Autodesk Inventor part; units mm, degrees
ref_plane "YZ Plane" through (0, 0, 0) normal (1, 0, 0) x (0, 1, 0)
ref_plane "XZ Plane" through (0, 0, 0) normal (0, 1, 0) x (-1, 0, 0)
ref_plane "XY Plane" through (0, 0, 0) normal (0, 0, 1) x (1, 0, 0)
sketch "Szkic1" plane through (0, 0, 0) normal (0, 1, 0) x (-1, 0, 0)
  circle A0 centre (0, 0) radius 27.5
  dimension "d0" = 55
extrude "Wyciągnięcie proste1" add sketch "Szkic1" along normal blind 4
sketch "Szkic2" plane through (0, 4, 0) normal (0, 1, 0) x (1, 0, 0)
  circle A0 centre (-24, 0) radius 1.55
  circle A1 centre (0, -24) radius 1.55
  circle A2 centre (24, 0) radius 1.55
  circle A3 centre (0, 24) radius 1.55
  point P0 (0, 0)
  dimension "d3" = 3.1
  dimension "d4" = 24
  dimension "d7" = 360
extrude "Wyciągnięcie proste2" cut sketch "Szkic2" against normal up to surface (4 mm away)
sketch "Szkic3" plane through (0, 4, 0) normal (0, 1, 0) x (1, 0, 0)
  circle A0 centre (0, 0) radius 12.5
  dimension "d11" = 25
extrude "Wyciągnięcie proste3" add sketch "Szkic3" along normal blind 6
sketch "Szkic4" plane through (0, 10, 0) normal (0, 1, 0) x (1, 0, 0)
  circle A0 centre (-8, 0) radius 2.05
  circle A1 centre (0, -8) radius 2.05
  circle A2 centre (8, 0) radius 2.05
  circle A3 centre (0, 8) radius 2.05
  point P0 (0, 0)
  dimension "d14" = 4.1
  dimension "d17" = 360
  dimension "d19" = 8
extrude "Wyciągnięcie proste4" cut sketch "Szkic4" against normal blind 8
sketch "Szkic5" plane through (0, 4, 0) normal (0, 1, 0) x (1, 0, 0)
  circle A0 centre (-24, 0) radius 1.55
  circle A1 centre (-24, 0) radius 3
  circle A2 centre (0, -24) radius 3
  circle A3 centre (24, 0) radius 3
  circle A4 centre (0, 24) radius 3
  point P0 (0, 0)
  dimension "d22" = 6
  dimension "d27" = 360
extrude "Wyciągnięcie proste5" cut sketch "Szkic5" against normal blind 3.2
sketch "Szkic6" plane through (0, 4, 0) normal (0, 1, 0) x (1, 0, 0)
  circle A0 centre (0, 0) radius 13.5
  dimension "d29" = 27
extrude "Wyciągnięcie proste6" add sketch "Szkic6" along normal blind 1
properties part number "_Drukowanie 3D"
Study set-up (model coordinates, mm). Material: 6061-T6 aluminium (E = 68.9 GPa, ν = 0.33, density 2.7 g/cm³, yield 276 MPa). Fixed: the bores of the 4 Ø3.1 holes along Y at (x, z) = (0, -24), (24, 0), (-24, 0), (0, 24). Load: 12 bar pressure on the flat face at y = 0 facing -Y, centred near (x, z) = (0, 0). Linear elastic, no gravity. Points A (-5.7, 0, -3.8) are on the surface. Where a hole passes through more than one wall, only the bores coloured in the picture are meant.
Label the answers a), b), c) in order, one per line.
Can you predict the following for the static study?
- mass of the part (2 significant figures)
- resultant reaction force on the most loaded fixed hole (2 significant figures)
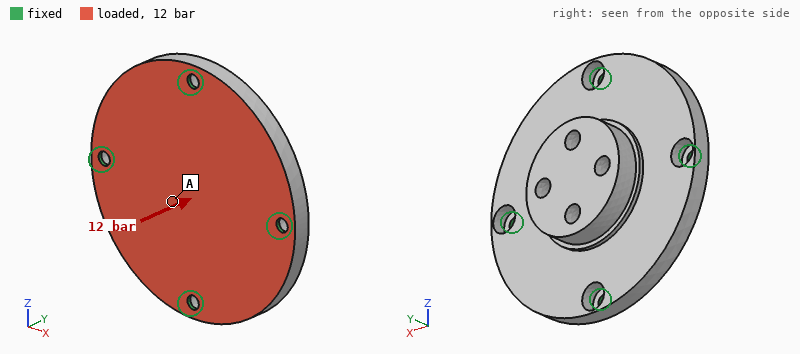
a) 32 g
b) 880 N
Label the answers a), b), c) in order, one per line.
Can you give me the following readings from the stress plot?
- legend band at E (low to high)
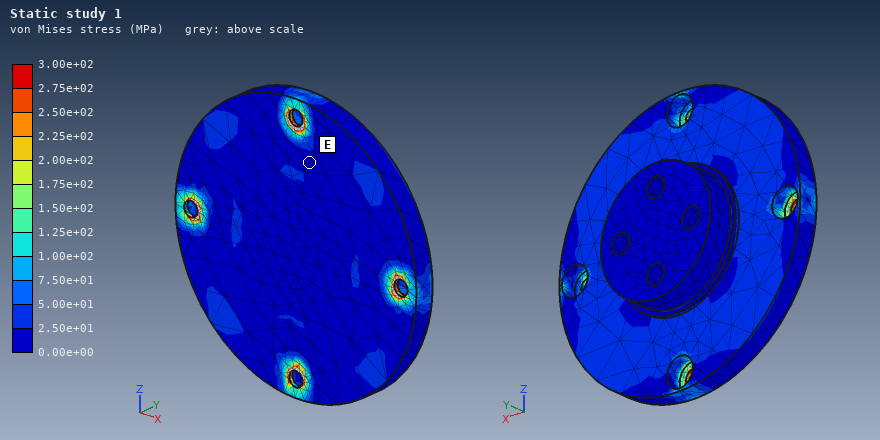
a) 0.00e+00 to 2.50e+01 MPa
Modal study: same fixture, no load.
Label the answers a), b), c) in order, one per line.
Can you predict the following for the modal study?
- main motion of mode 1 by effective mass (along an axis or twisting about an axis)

a) along Y
